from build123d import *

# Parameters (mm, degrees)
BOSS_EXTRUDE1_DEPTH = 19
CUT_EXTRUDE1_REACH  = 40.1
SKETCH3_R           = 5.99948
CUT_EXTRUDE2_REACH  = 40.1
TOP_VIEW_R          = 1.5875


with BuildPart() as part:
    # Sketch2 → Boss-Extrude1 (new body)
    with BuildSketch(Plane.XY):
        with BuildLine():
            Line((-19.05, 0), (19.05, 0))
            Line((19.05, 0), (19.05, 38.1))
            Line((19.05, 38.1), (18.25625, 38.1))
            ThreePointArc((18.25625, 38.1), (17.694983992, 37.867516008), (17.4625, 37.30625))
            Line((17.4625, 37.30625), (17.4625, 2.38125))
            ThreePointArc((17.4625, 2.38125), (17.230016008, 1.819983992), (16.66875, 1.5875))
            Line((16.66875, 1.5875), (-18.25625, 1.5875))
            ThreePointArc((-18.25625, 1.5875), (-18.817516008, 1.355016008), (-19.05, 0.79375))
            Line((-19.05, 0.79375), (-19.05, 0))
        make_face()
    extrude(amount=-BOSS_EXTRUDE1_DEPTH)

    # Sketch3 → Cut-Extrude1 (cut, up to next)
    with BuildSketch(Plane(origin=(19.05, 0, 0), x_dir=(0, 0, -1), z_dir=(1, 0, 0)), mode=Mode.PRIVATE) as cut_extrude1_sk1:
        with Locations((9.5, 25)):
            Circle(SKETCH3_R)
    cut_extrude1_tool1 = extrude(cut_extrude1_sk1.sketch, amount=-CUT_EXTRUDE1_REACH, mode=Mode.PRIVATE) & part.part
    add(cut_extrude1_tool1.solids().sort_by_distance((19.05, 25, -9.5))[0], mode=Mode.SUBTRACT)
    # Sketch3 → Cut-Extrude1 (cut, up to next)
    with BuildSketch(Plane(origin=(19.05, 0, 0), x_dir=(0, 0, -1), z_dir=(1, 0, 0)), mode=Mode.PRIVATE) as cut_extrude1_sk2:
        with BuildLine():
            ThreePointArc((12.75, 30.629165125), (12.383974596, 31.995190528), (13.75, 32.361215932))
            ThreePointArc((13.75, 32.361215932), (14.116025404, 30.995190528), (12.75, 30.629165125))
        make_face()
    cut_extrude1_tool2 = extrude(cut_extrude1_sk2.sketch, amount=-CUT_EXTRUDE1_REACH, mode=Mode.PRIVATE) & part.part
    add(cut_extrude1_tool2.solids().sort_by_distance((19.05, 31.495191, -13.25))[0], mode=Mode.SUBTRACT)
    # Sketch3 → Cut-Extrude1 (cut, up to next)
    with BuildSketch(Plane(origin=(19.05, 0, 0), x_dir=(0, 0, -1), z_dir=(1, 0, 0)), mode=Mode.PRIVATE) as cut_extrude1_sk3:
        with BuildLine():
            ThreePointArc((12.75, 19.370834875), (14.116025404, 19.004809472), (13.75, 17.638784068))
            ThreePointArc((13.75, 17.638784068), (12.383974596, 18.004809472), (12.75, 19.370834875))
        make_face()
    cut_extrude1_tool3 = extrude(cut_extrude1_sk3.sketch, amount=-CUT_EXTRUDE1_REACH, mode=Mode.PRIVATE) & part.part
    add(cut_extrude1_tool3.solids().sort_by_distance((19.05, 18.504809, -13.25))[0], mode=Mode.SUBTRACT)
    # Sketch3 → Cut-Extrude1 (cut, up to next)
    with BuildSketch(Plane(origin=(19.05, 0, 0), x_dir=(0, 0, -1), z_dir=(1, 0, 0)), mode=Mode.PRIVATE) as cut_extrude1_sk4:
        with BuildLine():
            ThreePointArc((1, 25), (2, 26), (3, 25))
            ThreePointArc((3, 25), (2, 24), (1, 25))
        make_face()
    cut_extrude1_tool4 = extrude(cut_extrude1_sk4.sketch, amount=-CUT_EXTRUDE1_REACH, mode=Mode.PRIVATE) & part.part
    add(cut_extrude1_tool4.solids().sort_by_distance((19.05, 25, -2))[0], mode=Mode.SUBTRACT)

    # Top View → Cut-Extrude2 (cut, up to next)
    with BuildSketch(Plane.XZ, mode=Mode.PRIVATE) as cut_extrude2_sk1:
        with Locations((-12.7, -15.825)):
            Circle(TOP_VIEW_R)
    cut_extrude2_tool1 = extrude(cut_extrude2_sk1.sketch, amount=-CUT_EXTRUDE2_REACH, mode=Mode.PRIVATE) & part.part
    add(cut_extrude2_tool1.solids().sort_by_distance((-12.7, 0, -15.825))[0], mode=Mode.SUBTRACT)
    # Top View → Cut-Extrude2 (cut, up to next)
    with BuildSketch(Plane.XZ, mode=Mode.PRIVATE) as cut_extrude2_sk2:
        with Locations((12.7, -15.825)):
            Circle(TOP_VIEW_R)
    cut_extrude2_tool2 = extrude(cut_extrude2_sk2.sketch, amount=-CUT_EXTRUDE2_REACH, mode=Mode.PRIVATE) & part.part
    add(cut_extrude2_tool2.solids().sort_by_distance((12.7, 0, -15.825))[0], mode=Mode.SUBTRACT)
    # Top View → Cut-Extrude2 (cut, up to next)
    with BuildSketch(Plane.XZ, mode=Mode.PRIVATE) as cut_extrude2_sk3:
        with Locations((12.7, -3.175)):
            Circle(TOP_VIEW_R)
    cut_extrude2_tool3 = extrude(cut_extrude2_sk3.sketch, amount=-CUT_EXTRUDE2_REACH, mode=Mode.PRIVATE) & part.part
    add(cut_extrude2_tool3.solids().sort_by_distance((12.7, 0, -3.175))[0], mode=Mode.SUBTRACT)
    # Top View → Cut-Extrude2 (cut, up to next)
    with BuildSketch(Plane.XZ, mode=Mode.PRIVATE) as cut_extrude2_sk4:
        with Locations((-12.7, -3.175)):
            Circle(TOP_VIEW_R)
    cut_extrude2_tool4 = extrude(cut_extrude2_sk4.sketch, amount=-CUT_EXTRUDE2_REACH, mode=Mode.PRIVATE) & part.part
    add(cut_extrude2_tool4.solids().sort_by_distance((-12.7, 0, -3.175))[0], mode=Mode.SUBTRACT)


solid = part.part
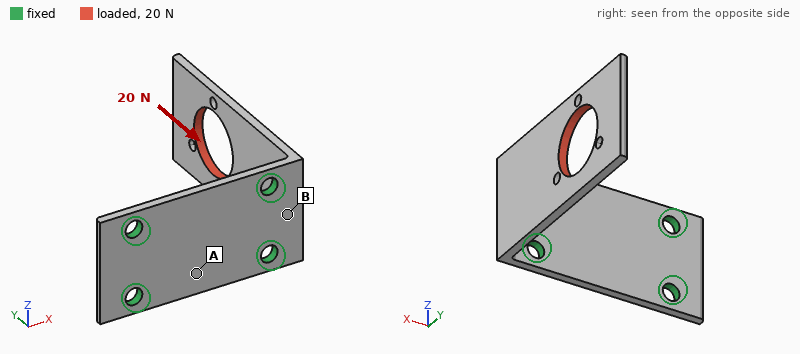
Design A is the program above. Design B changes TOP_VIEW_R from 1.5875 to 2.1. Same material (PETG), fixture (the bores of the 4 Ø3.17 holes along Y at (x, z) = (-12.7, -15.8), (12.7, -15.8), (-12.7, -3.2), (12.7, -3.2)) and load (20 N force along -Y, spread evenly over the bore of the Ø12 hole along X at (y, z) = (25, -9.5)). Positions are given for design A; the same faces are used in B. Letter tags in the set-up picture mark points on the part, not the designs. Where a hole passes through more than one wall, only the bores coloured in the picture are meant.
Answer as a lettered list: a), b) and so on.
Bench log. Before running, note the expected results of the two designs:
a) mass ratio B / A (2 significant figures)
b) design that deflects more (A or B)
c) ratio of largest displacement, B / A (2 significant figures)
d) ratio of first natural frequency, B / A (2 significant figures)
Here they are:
a) 0.98
b) A
c) 0.76
d) 1.0
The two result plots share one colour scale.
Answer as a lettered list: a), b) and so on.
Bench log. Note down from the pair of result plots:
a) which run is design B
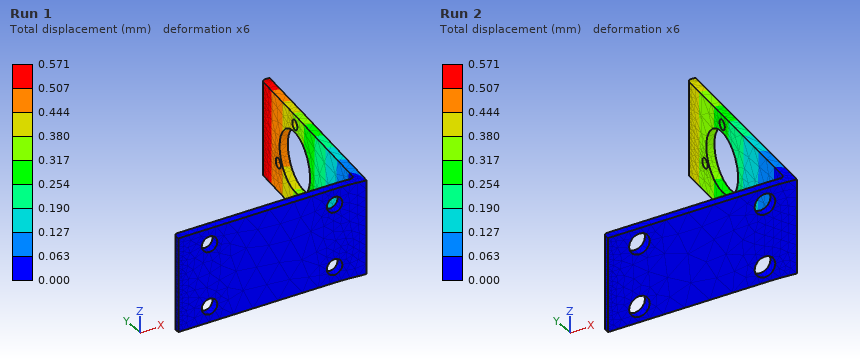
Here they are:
a) Run 2
